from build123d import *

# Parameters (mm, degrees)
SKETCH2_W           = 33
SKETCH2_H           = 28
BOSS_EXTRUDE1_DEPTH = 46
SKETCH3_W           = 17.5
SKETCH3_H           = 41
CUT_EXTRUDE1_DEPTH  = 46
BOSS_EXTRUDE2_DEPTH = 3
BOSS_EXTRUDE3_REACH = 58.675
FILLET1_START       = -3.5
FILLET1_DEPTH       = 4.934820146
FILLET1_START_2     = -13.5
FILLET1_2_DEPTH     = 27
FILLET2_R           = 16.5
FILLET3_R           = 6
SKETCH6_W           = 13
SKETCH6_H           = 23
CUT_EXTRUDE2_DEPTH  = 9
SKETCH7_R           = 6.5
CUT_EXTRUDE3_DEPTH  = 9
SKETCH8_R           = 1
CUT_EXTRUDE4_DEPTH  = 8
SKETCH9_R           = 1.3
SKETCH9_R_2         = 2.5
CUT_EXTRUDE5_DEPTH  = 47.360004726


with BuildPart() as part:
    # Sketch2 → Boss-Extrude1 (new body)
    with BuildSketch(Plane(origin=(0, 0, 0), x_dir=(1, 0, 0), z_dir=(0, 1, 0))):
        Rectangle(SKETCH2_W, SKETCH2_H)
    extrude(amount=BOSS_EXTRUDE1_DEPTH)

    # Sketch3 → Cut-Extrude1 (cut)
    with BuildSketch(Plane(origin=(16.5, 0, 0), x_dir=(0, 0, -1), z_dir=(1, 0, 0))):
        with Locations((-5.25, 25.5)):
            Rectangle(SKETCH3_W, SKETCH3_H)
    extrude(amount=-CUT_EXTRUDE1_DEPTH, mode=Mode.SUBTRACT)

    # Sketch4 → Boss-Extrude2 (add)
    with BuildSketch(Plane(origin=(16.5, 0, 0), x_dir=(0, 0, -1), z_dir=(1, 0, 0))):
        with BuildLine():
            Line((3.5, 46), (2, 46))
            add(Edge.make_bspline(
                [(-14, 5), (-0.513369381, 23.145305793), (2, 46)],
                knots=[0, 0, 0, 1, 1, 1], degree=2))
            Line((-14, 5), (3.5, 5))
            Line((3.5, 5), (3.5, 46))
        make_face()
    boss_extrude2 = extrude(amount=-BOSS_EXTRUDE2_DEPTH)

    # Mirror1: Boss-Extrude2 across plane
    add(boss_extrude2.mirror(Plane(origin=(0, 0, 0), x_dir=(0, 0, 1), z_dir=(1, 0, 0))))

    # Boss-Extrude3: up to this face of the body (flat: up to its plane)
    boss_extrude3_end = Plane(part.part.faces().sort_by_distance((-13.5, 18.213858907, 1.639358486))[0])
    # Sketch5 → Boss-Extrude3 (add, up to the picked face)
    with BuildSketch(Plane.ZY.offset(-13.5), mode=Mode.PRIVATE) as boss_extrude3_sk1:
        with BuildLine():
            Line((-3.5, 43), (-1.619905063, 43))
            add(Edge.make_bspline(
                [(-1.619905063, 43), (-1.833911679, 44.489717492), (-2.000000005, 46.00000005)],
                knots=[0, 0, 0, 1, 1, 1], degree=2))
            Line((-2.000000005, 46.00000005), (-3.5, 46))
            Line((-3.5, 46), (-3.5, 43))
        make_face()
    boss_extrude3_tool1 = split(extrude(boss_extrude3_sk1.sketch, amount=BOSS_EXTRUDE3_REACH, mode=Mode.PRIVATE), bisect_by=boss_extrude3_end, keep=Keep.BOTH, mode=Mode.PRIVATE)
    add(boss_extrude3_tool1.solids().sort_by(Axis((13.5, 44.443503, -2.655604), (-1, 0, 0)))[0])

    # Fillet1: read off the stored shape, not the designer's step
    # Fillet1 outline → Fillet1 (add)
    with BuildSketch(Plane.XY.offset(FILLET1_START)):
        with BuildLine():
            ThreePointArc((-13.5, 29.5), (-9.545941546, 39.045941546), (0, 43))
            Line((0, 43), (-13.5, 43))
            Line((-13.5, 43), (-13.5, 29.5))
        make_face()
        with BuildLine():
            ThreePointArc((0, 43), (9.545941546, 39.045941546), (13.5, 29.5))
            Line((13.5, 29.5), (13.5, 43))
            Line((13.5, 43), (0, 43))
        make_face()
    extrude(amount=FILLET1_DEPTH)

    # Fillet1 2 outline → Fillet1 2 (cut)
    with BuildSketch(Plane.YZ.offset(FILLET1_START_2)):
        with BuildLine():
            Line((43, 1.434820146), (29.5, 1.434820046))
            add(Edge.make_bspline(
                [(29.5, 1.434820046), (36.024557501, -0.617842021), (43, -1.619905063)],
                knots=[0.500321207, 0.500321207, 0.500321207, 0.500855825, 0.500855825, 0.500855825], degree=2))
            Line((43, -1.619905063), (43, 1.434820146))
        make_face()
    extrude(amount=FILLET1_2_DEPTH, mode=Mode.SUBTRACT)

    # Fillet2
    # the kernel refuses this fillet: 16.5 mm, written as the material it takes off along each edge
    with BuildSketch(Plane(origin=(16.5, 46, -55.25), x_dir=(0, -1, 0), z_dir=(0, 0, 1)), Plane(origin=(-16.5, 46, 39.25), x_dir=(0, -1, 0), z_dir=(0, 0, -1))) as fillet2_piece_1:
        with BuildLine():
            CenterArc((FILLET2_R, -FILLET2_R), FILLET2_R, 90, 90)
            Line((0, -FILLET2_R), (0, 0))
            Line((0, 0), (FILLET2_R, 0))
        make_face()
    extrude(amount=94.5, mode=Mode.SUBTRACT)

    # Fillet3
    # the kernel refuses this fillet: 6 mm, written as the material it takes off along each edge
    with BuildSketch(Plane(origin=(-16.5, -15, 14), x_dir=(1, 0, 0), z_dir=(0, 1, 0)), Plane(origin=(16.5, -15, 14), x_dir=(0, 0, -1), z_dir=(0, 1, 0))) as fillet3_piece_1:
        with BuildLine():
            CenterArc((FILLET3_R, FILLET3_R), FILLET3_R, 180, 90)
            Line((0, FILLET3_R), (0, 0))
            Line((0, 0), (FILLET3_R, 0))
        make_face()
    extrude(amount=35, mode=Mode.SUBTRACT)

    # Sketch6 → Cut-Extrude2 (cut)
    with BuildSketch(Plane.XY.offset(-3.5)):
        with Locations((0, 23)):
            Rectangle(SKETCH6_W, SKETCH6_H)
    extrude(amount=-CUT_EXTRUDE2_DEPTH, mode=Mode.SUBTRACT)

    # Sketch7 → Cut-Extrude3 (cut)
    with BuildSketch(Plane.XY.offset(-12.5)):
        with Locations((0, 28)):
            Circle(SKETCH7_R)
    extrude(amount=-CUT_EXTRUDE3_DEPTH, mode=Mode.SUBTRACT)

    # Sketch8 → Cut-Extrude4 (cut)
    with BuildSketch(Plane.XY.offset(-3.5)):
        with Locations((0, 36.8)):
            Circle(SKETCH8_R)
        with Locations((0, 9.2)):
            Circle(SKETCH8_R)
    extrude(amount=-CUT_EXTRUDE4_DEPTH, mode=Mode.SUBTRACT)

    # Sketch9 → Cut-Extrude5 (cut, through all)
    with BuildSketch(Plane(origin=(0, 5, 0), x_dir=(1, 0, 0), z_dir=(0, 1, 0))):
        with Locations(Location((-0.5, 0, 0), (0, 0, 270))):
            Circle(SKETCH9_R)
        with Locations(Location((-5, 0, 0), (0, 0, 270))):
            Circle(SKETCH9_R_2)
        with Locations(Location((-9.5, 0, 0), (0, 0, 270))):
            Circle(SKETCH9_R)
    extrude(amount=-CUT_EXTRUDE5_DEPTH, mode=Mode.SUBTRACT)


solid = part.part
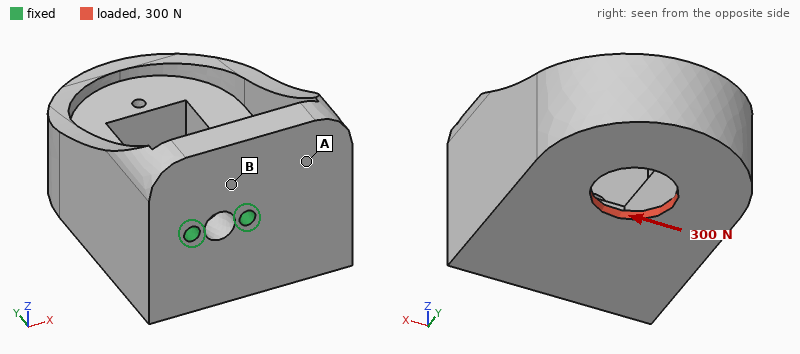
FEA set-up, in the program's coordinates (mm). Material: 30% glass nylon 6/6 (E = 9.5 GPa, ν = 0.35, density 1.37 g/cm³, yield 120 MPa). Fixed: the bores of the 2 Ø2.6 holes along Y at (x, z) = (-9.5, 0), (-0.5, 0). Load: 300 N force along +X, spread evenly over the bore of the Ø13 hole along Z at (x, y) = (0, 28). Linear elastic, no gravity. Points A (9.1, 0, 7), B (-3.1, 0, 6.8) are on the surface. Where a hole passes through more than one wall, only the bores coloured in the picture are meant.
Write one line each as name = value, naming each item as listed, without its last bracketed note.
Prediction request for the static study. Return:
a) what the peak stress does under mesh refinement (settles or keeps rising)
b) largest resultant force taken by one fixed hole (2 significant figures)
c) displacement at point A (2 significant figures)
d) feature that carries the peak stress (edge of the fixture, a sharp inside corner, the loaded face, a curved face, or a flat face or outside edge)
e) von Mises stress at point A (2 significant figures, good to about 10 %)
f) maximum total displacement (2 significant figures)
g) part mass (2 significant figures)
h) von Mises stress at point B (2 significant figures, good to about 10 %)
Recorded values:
what the peak stress does under mesh refinement = keeps rising
largest resultant force taken by one fixed hole = 640 N
displacement at point A = 0.053 mm
feature that carries the peak stress = edge of the fixture
von Mises stress at point A = 4.6 MPa
maximum total displacement = 0.24 mm
part mass = 22 g
von Mises stress at point B = 8.0 MPa
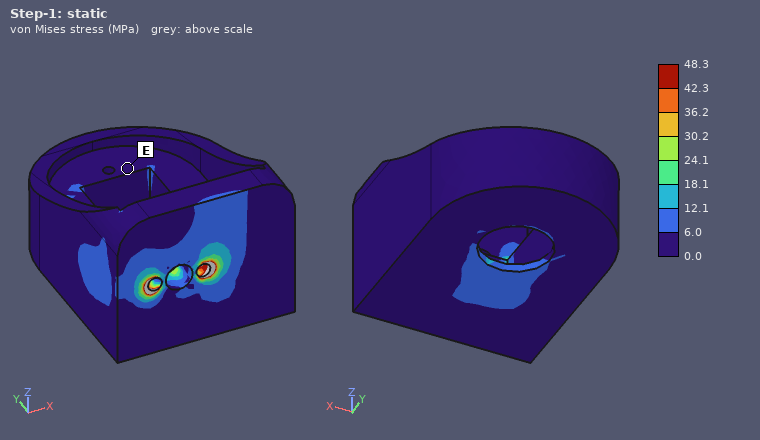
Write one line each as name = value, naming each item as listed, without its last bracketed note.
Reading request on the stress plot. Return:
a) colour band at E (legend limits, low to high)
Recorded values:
colour band at E = 0.0 to 6.0 MPa
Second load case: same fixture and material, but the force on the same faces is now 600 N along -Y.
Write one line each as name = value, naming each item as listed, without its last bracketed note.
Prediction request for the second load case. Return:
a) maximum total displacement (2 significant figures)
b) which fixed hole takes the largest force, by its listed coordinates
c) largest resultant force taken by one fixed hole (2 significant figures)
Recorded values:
maximum total displacement = 0.53 mm
which fixed hole takes the largest force, by its listed coordinates = (-0.5, 0)
largest resultant force taken by one fixed hole = 490 N
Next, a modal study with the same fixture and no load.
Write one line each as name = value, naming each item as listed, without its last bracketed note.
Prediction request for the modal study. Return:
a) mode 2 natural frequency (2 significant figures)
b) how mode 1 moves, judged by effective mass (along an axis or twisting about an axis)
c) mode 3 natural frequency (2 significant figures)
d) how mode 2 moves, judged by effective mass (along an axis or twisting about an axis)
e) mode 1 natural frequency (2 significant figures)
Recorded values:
mode 2 natural frequency = 1700 Hz
how mode 1 moves, judged by effective mass = along Z
mode 3 natural frequency = 3900 Hz
how mode 2 moves, judged by effective mass = along X
mode 1 natural frequency = 1200 Hz
